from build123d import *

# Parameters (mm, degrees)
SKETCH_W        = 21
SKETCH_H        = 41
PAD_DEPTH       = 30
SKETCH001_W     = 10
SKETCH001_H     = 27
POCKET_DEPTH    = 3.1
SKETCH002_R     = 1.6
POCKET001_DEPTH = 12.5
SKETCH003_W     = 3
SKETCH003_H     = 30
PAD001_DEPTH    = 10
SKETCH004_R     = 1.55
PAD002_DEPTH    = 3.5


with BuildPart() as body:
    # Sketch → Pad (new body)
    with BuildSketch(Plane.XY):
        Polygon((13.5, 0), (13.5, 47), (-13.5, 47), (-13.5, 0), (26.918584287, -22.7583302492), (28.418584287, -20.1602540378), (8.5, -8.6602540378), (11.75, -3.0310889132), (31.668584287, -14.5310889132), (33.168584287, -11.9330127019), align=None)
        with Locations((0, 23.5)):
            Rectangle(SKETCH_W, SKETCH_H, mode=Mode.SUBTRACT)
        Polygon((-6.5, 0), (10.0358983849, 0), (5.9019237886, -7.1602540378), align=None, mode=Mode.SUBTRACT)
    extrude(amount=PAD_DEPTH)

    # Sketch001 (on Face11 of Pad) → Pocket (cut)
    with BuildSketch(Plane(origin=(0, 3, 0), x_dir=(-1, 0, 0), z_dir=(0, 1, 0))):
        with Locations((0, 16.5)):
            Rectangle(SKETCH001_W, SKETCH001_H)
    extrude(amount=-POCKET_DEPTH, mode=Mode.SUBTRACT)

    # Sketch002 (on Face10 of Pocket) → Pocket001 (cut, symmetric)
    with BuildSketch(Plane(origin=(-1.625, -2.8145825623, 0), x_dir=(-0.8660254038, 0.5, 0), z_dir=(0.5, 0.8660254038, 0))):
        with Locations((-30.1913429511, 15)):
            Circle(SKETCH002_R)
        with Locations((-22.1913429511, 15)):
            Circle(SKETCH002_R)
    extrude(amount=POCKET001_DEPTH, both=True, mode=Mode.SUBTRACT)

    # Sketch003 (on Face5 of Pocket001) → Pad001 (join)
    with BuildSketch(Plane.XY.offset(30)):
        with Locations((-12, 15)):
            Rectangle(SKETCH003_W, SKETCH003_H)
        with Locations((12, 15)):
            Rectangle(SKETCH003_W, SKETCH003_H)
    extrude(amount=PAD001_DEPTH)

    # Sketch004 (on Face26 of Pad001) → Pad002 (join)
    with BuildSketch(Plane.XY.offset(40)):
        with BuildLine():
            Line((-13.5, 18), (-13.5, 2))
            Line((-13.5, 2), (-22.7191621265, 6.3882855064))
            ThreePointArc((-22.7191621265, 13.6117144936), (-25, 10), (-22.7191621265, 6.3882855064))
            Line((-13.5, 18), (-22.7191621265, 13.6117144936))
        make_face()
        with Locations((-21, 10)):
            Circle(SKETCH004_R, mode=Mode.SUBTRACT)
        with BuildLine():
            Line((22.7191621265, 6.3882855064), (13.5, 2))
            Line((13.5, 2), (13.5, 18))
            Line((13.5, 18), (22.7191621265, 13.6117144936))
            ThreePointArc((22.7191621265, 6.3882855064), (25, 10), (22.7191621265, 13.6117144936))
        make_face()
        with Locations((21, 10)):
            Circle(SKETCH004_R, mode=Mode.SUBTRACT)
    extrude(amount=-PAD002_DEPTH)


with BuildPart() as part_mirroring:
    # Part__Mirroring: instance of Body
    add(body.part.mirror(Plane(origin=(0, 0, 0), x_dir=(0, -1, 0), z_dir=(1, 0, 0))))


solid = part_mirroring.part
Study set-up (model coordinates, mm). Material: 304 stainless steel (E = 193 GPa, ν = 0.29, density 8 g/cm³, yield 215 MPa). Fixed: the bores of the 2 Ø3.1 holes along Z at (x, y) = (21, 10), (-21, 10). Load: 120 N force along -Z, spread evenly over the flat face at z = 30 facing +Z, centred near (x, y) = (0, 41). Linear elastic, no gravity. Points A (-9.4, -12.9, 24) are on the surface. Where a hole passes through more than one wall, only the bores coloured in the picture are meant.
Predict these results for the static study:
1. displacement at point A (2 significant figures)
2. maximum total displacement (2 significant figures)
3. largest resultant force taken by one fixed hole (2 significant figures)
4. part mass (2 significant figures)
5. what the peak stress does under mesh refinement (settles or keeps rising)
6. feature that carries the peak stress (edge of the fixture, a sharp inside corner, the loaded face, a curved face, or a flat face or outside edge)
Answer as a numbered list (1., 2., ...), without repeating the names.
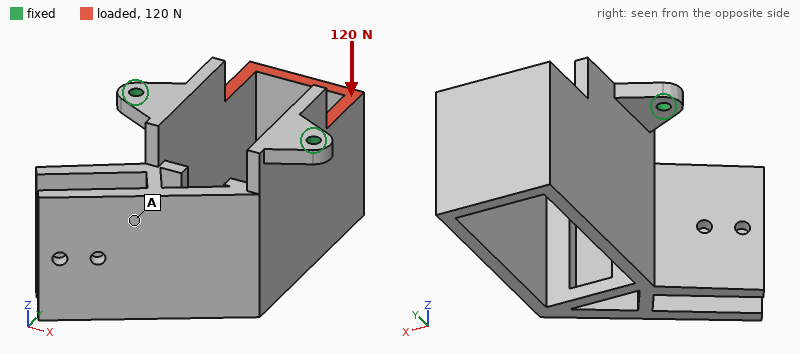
1. 31 µm
2. 65 µm
3. 60 N
4. 170 g
5. keeps rising
6. edge of the fixture
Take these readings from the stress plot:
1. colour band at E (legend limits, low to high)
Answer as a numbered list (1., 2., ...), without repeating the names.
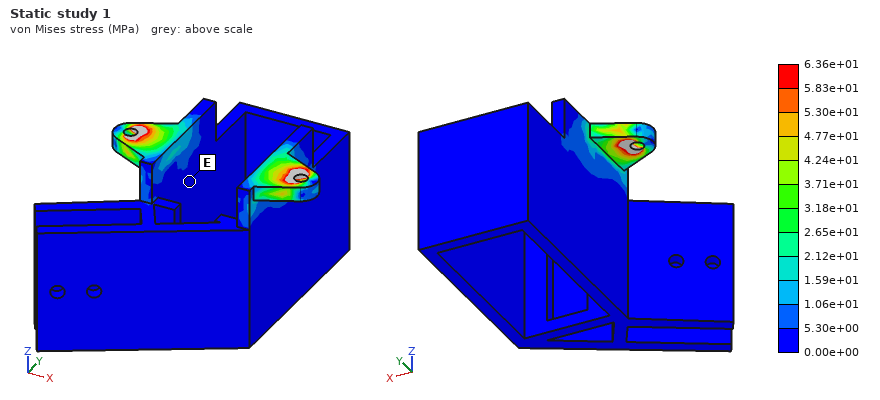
1. 0.00e+00 to 5.30e+00 MPa
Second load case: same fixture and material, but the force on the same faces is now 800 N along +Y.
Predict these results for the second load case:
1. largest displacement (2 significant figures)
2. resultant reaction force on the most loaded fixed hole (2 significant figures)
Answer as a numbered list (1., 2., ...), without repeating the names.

1. 0.12 mm
2. 400 N
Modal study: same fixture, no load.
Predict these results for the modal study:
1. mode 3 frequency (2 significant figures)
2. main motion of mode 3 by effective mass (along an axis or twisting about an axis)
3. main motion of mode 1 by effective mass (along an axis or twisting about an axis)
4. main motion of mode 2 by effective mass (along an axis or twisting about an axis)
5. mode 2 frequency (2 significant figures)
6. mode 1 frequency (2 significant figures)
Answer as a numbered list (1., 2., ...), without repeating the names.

1. 2600 Hz
2. along X
3. along Y
4. along X
5. 1600 Hz
6. 690 Hz
